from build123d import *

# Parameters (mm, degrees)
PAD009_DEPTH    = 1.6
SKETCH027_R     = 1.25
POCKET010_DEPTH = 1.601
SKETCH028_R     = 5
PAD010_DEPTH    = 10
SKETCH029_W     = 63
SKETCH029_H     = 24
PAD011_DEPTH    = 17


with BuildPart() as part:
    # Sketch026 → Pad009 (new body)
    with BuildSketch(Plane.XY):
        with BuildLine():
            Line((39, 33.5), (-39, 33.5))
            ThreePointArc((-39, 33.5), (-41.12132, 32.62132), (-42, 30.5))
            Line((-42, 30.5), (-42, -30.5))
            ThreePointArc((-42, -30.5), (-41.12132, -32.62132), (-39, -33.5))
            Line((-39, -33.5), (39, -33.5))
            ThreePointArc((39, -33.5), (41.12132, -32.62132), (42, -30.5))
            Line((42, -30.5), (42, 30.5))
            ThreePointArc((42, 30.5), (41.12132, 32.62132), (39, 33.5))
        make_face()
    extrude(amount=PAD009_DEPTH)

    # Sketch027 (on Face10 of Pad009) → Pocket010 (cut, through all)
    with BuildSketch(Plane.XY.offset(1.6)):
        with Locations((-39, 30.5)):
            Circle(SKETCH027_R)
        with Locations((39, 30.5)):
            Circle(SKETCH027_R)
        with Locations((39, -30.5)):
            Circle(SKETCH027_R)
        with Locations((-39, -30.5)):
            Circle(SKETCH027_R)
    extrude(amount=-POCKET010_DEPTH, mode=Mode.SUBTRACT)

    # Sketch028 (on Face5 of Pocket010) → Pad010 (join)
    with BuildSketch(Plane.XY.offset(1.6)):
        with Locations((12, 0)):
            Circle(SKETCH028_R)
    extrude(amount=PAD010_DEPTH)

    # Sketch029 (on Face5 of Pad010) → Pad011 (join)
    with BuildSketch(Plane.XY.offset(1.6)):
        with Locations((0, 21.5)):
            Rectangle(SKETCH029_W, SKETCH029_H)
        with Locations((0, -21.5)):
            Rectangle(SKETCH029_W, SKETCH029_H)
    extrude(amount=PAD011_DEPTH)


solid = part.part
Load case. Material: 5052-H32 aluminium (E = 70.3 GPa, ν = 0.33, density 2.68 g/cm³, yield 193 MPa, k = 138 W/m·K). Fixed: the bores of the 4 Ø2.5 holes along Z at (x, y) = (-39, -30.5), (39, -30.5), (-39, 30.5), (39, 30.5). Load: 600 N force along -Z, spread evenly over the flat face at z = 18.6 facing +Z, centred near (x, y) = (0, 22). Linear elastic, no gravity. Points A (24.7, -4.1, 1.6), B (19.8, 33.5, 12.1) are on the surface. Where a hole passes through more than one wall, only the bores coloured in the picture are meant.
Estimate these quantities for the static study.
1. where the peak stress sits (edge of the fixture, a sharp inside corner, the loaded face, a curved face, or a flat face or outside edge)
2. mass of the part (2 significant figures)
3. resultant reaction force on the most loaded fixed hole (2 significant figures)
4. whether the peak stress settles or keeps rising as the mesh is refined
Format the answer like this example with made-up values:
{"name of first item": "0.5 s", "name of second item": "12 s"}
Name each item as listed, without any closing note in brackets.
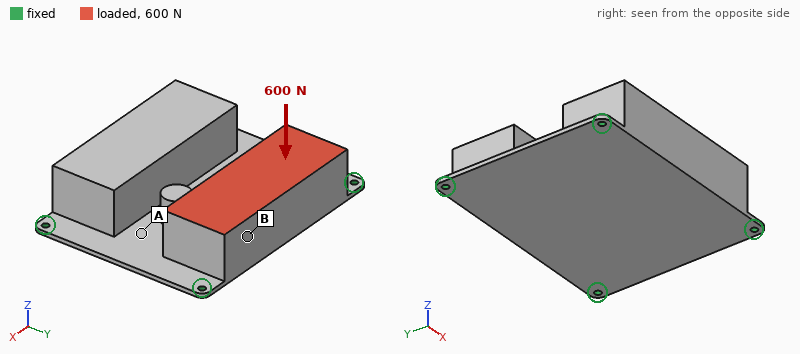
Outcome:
{"where the peak stress sits": "edge of the fixture", "mass of the part": "160 g", "resultant reaction force on the most loaded fixed hole": "300 N", "whether the peak stress settles or keeps rising as the mesh is refined": "keeps rising"}
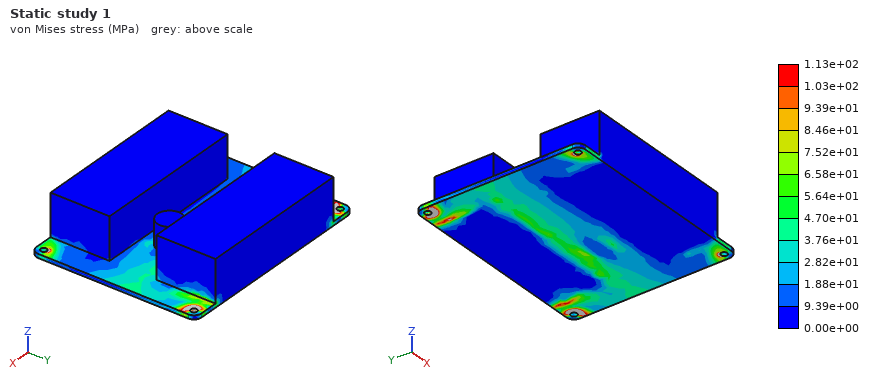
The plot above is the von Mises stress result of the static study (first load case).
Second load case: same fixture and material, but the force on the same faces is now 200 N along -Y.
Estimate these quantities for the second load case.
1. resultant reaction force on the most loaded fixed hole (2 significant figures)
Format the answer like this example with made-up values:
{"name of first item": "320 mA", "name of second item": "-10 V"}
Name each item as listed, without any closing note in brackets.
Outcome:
{"resultant reaction force on the most loaded fixed hole": "73 N"}
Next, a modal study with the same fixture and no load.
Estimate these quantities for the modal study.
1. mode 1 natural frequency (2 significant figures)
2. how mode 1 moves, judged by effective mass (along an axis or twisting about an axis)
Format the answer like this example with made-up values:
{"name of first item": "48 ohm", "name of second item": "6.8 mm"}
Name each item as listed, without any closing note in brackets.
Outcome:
{"mode 1 natural frequency": "720 Hz", "how mode 1 moves, judged by effective mass": "along Z"}
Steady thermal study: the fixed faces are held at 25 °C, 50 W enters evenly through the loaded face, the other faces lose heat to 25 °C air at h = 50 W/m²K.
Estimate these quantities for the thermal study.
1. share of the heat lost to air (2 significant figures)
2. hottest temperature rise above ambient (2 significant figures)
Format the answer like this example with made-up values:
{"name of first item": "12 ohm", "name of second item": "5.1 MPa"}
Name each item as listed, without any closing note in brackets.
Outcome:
{"share of the heat lost to air": "41 %", "hottest temperature rise above ambient": "44 K"}
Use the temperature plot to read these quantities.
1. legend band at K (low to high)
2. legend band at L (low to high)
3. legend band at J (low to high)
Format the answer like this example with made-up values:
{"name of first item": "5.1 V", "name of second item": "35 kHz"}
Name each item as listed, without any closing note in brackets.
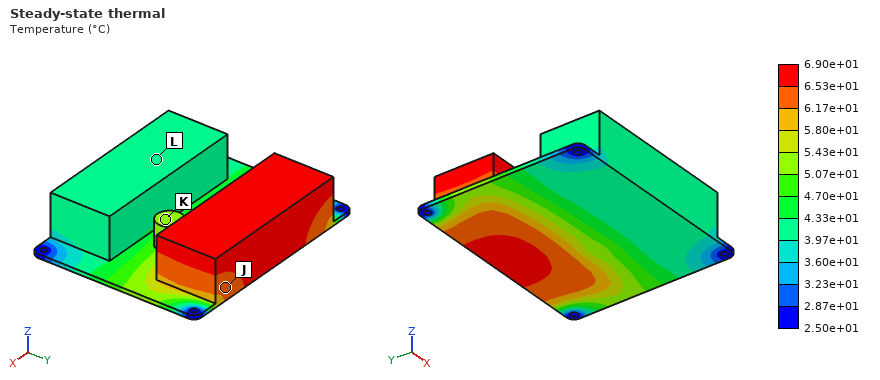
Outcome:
{"legend band at K": "5.07e+01 to 5.43e+01 °C", "legend band at L": "3.97e+01 to 4.33e+01 °C", "legend band at J": "6.17e+01 to 6.53e+01 °C"}
